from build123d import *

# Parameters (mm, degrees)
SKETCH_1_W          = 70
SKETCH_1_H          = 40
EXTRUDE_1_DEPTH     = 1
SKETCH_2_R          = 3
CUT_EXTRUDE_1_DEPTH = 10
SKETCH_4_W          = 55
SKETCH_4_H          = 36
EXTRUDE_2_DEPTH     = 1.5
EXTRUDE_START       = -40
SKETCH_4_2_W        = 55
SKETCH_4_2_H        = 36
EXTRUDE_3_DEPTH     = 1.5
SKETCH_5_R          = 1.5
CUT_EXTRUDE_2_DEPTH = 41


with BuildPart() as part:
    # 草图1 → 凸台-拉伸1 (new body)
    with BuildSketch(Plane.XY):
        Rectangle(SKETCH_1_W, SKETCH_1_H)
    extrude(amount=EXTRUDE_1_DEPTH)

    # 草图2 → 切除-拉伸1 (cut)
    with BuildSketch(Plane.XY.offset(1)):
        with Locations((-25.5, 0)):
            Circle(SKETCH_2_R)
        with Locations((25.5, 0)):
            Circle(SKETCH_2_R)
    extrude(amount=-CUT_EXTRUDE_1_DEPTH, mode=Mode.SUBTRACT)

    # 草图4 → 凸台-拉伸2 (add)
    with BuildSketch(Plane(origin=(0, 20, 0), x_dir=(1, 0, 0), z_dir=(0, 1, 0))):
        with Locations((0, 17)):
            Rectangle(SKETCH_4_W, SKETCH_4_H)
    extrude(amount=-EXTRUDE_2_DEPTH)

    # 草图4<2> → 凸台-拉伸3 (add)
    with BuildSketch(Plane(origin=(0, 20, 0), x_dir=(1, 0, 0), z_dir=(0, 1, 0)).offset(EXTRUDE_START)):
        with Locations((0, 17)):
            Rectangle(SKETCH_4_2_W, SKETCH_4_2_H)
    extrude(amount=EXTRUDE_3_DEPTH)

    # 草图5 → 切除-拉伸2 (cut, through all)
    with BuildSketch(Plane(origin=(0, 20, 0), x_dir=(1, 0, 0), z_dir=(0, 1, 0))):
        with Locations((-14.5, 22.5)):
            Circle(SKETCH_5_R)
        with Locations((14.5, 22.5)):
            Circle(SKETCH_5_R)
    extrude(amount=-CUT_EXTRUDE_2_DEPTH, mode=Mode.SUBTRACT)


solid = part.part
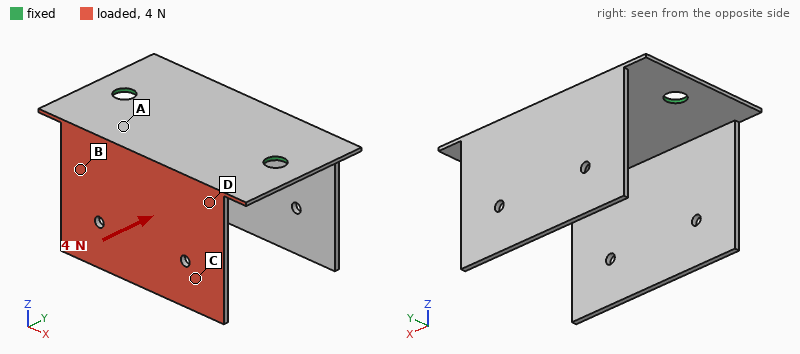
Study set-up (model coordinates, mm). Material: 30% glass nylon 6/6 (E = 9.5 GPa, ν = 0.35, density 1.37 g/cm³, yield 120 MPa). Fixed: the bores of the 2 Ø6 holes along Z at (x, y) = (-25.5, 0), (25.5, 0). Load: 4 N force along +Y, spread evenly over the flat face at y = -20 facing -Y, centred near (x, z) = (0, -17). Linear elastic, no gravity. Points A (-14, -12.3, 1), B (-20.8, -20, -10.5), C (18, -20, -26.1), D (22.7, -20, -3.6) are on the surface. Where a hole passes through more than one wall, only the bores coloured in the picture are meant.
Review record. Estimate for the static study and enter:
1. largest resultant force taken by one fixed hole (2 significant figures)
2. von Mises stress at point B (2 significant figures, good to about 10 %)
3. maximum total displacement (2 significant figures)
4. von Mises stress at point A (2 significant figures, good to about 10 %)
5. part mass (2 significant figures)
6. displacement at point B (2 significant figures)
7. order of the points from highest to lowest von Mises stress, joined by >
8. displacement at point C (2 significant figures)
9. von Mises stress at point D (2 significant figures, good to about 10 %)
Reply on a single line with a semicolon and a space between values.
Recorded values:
2.0 N; 1.5 MPa; 0.91 mm; 5.5 MPa; 12 g; 0.33 mm; A > D > B > C; 0.68 mm; 2.2 MPa
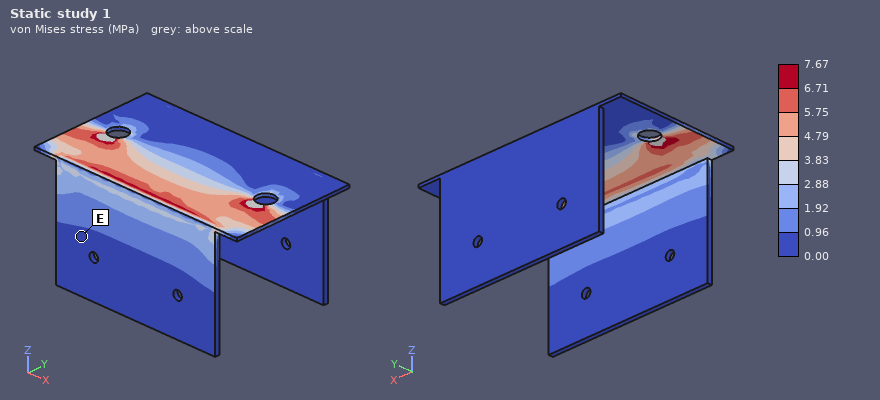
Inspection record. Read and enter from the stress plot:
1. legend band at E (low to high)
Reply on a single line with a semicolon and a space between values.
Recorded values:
0.00 to 0.96 MPa
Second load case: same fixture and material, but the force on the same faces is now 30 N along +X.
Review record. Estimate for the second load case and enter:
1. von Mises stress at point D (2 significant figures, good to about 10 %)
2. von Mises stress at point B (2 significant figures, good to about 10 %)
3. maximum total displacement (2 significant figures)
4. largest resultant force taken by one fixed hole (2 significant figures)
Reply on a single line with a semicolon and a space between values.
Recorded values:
8.9 MPa; 4.3 MPa; 0.81 mm; 21 N
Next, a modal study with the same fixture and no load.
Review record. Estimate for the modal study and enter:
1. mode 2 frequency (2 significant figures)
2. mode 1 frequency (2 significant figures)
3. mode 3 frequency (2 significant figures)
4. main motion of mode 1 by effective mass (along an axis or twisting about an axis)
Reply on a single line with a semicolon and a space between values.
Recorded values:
190 Hz; 180 Hz; 480 Hz; along Y
